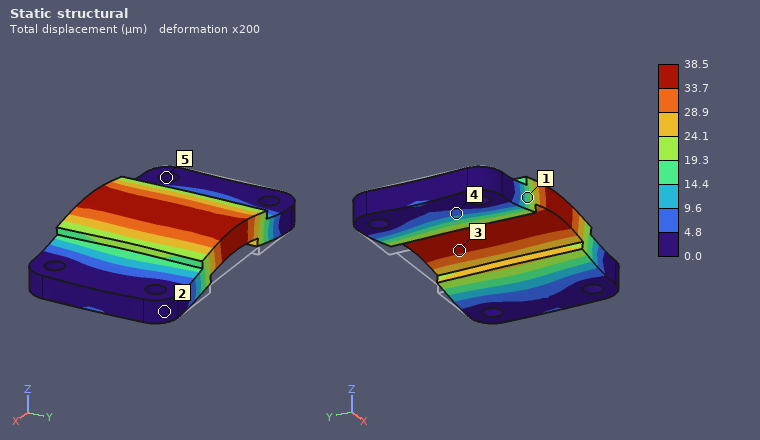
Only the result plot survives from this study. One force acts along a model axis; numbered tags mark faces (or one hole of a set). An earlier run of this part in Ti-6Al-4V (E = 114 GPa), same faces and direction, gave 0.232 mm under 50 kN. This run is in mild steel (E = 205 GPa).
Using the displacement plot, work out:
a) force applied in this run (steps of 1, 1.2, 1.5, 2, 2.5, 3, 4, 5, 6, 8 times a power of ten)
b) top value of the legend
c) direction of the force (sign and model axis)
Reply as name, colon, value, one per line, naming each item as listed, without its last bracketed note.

force applied in this run: 15 kN
top value of the legend: 38.5 µm
direction of the force: +Z
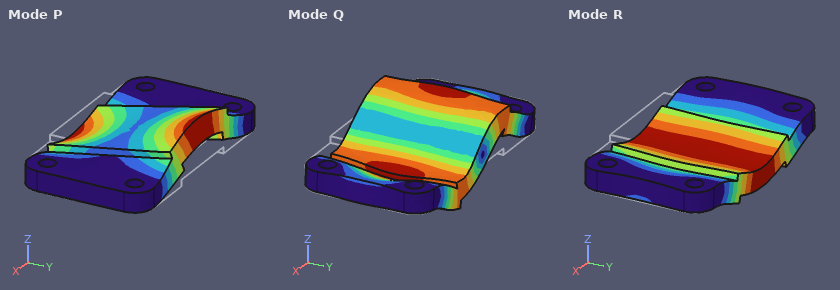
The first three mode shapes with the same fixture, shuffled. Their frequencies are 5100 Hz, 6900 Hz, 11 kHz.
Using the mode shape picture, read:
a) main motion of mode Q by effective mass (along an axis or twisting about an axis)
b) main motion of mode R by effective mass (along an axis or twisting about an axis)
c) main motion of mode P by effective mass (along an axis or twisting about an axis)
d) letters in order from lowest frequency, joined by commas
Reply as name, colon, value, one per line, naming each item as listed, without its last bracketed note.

main motion of mode Q by effective mass: twisting about Y
main motion of mode R by effective mass: along Z
main motion of mode P by effective mass: twisting about X
letters in order from lowest frequency, joined by commas: R, P, Q
